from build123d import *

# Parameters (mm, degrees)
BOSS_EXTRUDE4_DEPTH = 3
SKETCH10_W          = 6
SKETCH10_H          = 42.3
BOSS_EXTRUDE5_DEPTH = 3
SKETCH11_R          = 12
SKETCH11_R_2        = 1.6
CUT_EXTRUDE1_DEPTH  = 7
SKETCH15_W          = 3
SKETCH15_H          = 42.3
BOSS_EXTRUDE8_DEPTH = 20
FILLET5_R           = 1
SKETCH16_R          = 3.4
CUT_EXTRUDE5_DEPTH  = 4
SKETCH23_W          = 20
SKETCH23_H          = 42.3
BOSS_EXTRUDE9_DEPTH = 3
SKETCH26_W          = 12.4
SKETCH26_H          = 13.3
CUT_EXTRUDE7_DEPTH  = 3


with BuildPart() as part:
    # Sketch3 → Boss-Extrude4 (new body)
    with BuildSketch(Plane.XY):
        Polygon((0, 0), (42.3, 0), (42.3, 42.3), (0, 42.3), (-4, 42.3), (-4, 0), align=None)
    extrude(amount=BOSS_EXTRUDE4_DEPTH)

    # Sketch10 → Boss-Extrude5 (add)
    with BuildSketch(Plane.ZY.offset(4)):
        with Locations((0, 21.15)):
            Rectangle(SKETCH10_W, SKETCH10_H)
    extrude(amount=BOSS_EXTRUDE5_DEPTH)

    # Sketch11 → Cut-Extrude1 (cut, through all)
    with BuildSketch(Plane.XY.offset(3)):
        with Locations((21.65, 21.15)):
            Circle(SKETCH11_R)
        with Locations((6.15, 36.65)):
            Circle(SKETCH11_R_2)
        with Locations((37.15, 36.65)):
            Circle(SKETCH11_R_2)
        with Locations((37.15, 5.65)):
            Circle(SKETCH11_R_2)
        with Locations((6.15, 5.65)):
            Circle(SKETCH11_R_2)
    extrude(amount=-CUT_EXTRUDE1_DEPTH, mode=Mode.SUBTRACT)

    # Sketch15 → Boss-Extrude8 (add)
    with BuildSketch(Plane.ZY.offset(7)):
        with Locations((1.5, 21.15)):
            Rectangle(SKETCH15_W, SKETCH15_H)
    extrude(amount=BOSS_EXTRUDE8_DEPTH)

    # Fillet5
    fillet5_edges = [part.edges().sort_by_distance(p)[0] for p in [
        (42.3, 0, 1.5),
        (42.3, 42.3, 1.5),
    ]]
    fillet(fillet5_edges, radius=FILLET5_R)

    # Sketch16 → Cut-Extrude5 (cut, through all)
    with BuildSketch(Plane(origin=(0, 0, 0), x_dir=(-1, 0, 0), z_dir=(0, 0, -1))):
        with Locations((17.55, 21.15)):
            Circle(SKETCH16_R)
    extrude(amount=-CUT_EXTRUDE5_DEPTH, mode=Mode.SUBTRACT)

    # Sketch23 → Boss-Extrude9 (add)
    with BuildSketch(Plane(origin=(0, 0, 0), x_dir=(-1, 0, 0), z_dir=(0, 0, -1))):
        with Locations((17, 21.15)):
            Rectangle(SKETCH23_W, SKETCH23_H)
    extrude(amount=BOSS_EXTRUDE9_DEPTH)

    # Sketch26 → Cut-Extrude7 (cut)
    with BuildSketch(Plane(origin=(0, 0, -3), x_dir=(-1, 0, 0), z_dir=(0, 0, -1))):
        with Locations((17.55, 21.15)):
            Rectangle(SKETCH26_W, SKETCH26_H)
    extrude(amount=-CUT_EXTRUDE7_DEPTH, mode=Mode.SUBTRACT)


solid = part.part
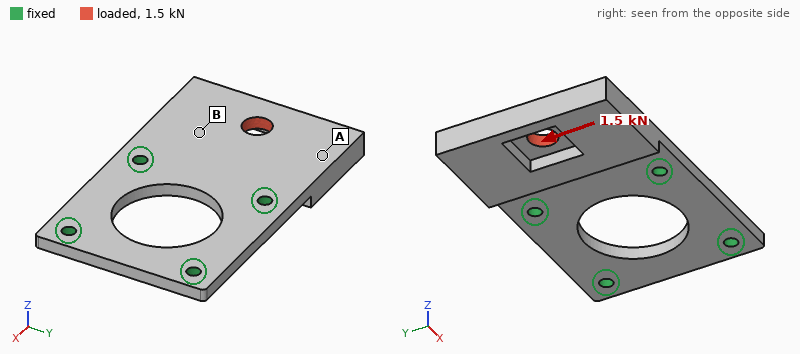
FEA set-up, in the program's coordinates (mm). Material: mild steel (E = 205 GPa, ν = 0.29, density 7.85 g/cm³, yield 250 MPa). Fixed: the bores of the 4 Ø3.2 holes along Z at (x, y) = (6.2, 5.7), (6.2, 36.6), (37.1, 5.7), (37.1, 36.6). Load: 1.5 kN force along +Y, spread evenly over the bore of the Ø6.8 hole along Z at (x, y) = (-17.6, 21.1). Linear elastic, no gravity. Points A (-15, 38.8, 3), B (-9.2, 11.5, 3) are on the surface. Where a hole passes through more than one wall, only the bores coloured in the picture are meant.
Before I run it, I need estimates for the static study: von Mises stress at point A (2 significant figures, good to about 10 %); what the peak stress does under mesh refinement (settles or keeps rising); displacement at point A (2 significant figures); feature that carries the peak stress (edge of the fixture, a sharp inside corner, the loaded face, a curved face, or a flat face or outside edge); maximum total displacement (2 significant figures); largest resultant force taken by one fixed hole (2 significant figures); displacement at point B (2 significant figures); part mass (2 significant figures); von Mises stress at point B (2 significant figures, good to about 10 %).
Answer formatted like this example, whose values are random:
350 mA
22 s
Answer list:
11 MPa
keeps rising
6.9 µm
edge of the fixture
11 µm
1.3 kN
4.3 µm
76 g
25 MPa
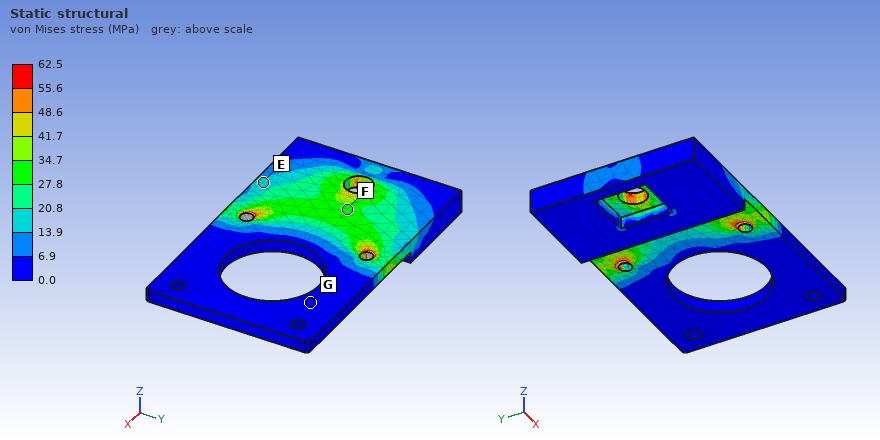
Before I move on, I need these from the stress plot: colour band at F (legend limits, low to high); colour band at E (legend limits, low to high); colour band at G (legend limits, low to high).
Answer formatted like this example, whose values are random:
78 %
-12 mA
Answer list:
27.8 to 34.7 MPa
13.9 to 20.8 MPa
0.0 to 6.9 MPa
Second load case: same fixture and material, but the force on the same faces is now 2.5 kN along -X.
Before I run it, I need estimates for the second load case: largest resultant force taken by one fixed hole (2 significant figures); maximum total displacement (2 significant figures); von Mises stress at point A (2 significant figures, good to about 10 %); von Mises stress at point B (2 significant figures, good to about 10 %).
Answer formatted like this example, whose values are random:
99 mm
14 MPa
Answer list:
1.2 kN
6.7 µm
12 MPa
28 MPa
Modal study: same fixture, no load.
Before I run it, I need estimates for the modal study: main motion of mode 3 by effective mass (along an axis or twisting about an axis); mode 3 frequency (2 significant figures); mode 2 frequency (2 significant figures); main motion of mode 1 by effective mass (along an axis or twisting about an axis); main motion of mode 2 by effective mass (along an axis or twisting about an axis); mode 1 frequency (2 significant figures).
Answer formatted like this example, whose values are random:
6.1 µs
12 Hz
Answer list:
along Y
13 kHz
5300 Hz
along Z
twisting about X
1700 Hz
